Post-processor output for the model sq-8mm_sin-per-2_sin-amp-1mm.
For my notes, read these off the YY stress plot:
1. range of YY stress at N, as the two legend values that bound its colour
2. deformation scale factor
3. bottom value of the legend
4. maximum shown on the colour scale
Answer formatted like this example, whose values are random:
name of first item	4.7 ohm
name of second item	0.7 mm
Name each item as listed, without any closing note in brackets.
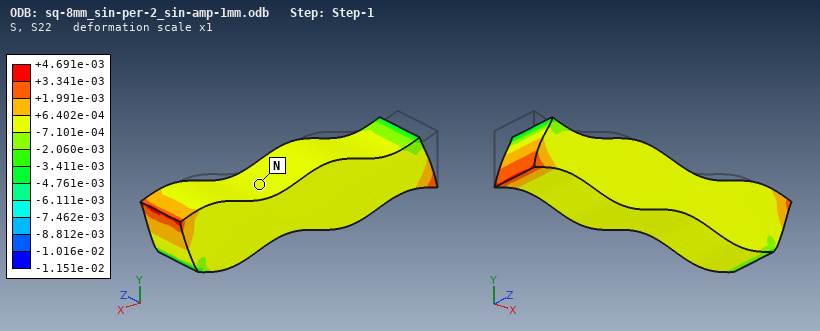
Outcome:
range of YY stress at N, as the two legend values that bound its colour	-7.101e-04 to +6.402e-04
deformation scale factor	1
bottom value of the legend	-1.151e-02
maximum shown on the colour scale	+4.691e-03
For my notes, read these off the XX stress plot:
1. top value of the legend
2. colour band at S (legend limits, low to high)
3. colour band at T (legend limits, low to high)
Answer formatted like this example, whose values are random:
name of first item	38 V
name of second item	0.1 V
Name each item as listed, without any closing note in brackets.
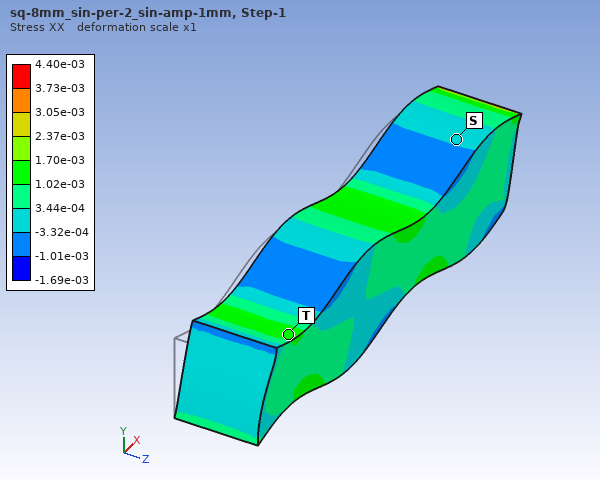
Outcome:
top value of the legend	4.40e-03
colour band at S	-3.32e-04 to 3.44e-04
colour band at T	1.02e-03 to 1.70e-03
